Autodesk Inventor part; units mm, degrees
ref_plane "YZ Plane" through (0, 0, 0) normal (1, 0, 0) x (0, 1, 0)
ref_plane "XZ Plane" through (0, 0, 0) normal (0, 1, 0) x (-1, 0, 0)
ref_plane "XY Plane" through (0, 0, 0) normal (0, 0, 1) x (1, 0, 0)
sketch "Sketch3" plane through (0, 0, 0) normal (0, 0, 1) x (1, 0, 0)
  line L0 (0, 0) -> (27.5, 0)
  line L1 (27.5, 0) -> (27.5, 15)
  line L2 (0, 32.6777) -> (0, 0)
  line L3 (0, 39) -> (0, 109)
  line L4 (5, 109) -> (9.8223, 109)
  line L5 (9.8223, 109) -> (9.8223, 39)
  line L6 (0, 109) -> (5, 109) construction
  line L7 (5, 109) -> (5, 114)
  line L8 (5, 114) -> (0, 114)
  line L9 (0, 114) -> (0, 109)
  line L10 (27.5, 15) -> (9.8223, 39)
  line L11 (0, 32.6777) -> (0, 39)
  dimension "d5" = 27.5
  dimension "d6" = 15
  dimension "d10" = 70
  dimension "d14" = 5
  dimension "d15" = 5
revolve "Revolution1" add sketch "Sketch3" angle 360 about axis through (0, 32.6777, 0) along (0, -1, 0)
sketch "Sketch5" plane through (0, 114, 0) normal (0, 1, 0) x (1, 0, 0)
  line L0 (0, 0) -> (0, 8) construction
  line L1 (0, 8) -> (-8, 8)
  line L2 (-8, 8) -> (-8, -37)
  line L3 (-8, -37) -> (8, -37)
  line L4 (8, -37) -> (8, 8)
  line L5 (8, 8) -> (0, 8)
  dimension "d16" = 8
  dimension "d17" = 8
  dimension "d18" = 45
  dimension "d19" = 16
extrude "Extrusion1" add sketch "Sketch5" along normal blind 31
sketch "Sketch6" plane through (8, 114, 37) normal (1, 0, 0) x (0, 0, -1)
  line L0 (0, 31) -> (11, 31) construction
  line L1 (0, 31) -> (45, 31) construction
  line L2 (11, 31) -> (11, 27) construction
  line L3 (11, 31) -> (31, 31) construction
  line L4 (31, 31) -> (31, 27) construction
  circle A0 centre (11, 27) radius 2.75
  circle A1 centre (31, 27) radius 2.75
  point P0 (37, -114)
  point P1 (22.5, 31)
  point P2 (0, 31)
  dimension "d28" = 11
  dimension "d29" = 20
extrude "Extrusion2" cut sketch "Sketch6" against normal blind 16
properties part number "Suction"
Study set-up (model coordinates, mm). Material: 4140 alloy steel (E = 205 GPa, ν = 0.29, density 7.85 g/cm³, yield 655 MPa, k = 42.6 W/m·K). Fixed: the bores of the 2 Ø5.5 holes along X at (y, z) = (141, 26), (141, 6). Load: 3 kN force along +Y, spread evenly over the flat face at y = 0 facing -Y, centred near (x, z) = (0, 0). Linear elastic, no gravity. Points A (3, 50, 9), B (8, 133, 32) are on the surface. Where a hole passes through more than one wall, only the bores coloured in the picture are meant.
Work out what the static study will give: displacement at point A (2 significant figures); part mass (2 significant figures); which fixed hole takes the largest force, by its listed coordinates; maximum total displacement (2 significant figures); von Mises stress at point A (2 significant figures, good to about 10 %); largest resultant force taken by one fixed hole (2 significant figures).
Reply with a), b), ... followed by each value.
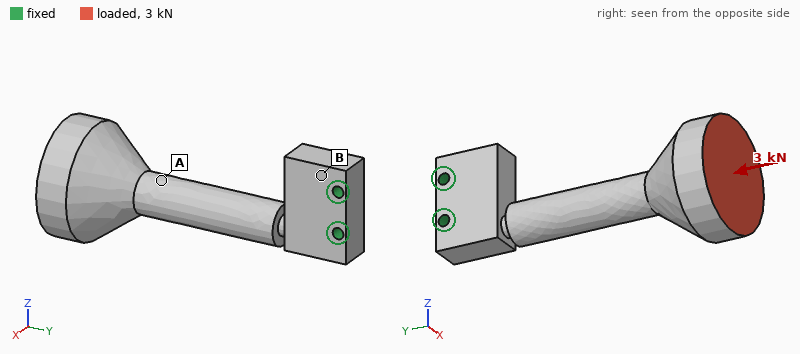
a) 9.2 µm
b) 840 g
c) (141, 6)
d) 15 µm
e) 10.0 MPa
f) 3.5 kN
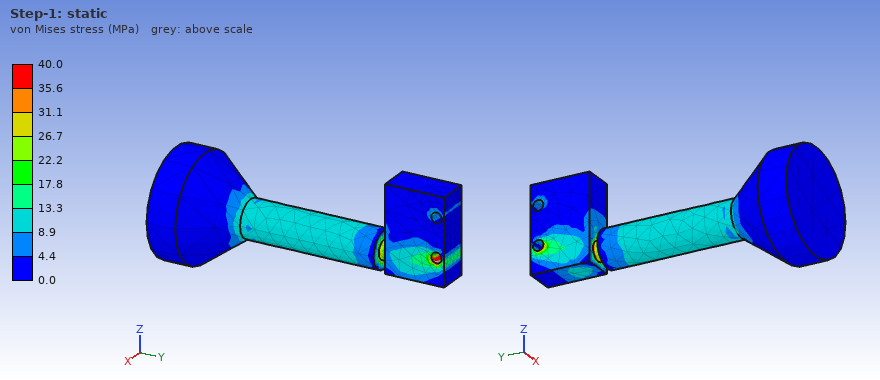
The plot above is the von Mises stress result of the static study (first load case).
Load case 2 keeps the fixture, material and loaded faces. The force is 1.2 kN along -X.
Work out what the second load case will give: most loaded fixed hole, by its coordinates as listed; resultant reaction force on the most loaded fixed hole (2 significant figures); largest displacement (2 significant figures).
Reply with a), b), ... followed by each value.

a) (141, 6)
b) 730 N
c) 2.0 mm
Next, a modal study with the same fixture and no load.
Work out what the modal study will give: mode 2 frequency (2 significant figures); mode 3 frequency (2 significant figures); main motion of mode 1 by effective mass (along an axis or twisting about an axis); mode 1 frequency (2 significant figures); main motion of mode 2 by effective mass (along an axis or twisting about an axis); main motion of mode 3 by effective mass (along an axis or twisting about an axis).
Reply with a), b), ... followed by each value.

a) 210 Hz
b) 950 Hz
c) along X
d) 200 Hz
e) along Z
f) twisting about Y
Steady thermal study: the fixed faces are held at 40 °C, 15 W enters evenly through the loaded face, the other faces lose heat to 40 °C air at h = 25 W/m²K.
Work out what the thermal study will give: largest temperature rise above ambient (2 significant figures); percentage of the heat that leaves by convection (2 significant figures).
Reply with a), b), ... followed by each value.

a) 53 K
b) 75 %
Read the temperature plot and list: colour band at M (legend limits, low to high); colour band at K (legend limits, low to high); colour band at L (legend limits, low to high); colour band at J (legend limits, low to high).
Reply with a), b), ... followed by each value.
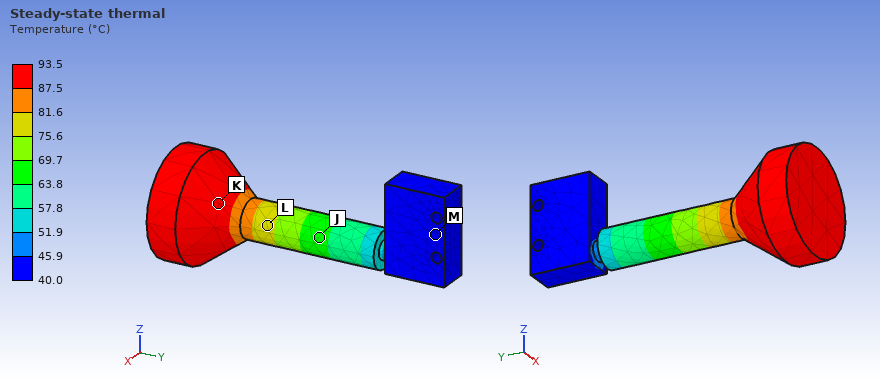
a) 40.0 to 45.9 °C
b) 87.5 to 93.5 °C
c) 75.6 to 81.6 °C
d) 63.8 to 69.7 °C
